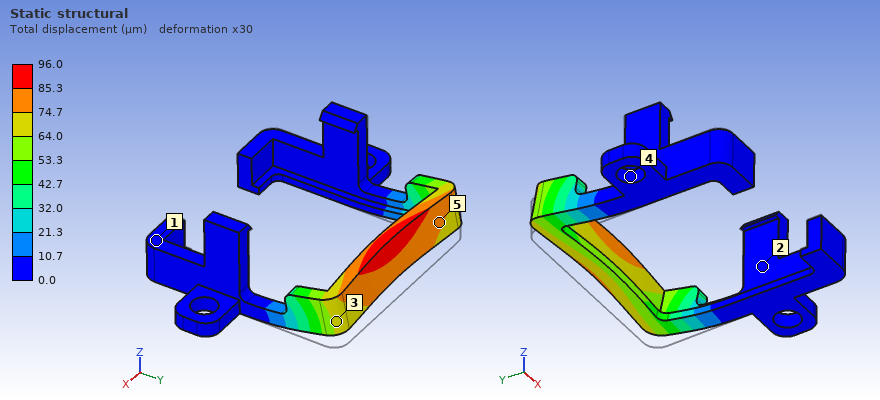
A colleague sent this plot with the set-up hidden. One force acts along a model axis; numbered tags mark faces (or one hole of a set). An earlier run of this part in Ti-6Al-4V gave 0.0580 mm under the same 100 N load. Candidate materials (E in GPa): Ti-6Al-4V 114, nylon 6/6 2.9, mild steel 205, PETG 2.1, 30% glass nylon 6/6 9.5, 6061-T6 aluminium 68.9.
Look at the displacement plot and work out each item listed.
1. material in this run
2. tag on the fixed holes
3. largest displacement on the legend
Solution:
6061-T6 aluminium
4
96.0 µm
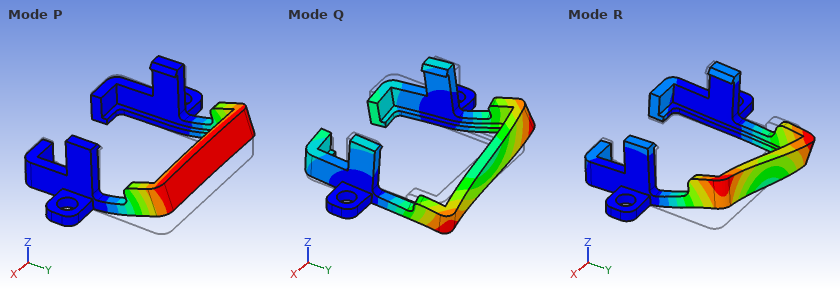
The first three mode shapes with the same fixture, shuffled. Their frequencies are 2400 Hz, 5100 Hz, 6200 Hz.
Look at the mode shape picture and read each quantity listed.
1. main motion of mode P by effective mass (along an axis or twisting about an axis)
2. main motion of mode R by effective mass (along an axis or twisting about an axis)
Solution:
along Z
along X
